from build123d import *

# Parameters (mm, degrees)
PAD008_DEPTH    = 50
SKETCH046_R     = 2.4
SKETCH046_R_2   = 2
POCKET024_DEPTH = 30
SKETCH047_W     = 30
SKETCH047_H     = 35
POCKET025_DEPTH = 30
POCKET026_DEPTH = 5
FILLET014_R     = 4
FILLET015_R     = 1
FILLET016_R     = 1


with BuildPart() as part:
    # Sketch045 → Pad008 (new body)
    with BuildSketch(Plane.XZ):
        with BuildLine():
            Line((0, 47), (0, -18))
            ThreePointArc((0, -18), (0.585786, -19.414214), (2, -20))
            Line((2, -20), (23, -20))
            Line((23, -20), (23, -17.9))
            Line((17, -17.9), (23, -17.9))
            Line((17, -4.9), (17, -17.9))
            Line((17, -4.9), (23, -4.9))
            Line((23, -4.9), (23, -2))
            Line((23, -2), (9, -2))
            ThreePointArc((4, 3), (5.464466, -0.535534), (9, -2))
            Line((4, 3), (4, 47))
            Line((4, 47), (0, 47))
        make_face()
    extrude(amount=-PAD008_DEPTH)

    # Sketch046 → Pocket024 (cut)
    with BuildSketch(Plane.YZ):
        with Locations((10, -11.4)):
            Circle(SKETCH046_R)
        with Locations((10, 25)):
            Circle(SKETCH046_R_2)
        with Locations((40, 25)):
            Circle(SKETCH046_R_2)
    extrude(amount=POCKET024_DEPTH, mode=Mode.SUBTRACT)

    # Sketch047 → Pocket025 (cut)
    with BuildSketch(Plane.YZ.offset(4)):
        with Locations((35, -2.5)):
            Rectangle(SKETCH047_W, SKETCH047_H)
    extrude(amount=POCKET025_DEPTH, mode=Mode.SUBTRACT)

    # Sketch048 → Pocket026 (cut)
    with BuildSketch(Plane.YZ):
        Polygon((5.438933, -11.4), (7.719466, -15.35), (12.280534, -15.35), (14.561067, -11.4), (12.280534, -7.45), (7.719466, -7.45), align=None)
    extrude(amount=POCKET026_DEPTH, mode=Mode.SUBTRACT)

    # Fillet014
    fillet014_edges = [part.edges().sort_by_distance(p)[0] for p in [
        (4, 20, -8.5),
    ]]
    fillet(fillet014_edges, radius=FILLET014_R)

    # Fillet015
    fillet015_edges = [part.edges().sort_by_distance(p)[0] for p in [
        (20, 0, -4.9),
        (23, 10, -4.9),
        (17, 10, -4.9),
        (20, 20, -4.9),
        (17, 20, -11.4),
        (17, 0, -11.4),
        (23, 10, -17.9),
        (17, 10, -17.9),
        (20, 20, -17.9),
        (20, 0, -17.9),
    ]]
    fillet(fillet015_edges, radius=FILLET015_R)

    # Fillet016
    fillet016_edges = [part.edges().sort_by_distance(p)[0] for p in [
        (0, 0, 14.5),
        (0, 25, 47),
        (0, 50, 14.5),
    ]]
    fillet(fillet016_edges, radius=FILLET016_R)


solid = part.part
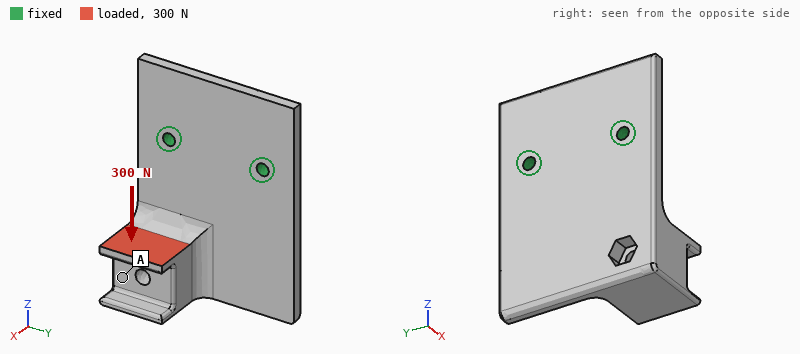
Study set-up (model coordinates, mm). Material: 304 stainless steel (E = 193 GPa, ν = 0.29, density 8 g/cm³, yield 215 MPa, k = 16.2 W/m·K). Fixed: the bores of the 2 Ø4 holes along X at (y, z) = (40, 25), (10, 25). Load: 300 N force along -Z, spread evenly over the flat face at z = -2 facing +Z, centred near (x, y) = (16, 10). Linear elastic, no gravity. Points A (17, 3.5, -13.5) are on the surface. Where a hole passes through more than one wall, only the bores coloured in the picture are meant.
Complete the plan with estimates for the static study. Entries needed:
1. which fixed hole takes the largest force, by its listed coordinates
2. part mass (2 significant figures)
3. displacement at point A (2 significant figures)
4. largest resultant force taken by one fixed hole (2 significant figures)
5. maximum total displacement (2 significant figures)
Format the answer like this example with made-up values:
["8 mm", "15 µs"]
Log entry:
["(10, 25)", "150 g", "73 µm", "290 N", "95 µm"]
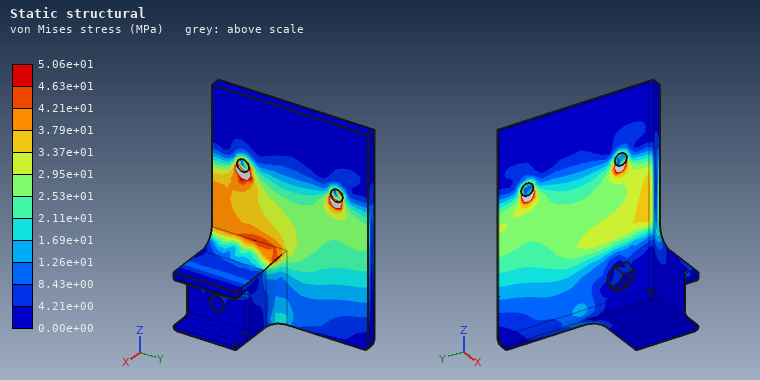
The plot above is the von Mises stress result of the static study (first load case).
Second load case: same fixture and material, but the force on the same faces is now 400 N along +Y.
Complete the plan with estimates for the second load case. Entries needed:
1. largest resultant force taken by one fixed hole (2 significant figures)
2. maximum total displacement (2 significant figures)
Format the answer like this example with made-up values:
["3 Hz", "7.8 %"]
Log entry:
["430 N", "43 µm"]
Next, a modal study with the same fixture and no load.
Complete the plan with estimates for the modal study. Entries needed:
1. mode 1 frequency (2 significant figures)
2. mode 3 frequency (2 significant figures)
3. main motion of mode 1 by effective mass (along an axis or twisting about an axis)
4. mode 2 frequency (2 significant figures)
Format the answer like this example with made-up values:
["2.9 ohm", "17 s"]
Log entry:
["980 Hz", "5500 Hz", "along X", "2700 Hz"]
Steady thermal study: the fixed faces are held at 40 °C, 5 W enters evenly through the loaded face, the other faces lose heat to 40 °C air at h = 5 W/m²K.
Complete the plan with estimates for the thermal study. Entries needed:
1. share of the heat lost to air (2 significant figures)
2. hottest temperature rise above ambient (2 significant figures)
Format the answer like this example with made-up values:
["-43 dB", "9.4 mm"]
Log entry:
["23 %", "76 K"]
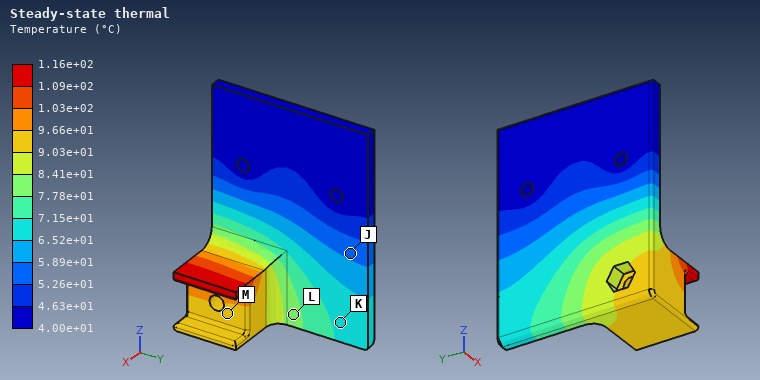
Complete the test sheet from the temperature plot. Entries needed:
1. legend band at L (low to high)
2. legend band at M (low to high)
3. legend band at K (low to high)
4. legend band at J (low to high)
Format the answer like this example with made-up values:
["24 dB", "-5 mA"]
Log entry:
["7.78e+01 to 8.41e+01 °C", "9.03e+01 to 9.66e+01 °C", "6.52e+01 to 7.15e+01 °C", "5.26e+01 to 5.89e+01 °C"]
